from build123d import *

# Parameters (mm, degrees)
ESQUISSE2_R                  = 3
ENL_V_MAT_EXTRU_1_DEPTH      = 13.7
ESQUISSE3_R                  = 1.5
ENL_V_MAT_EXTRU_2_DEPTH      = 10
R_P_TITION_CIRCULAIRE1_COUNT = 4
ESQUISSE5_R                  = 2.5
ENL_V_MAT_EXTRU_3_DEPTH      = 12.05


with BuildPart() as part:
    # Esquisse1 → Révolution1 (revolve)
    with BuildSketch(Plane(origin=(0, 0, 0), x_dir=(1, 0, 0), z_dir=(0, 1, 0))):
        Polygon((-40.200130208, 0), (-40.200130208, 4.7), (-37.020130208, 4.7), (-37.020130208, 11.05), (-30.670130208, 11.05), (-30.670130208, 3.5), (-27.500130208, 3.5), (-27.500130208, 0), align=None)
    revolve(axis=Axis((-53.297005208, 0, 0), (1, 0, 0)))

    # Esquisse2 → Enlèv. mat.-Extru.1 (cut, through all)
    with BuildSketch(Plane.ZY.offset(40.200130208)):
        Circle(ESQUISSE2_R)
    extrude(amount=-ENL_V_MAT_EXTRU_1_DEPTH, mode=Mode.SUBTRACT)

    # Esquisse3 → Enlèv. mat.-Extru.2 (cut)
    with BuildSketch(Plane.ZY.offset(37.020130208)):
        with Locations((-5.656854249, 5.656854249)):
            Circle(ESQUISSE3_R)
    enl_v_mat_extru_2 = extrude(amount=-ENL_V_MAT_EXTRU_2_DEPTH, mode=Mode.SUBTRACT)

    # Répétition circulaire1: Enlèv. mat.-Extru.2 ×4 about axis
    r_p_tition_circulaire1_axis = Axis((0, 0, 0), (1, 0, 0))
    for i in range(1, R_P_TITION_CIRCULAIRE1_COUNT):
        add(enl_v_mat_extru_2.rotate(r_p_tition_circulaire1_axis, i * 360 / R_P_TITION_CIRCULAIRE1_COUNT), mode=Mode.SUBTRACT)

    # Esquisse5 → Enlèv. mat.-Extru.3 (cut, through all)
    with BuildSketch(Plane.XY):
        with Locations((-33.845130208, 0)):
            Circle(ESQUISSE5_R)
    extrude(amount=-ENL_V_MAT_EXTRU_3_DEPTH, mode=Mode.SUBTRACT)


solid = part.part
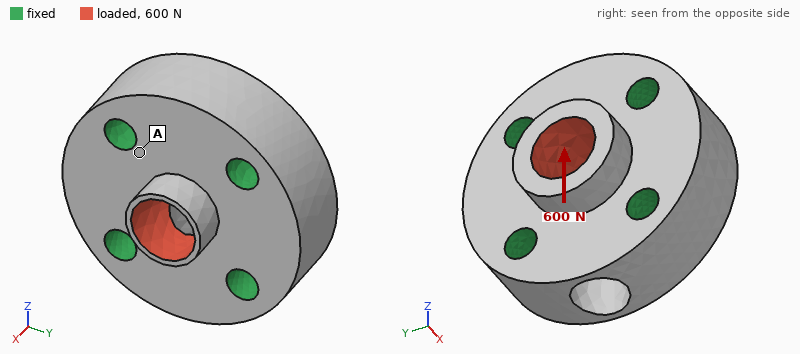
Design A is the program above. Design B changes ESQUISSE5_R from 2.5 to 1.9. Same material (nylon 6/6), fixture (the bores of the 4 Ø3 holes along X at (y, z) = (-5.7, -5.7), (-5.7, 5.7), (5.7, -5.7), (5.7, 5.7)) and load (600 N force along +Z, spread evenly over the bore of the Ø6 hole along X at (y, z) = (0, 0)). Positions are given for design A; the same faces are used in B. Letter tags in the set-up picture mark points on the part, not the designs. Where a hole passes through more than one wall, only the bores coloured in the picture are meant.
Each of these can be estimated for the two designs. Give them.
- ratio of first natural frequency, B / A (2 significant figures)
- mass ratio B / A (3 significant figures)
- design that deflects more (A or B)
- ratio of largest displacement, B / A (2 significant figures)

1.0
1.03
A
0.85
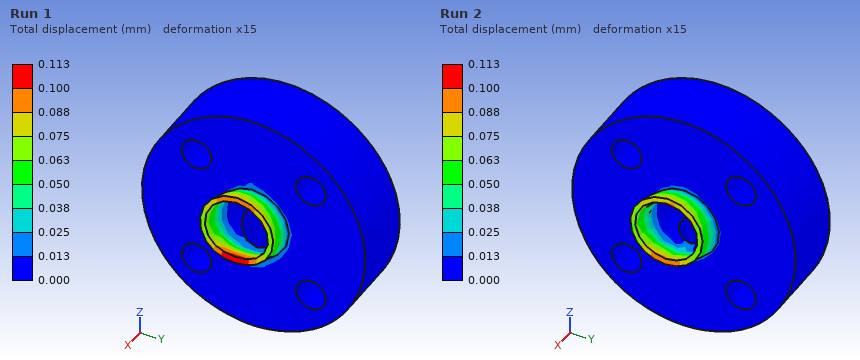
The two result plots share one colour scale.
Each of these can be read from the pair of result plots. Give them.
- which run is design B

Run 2
